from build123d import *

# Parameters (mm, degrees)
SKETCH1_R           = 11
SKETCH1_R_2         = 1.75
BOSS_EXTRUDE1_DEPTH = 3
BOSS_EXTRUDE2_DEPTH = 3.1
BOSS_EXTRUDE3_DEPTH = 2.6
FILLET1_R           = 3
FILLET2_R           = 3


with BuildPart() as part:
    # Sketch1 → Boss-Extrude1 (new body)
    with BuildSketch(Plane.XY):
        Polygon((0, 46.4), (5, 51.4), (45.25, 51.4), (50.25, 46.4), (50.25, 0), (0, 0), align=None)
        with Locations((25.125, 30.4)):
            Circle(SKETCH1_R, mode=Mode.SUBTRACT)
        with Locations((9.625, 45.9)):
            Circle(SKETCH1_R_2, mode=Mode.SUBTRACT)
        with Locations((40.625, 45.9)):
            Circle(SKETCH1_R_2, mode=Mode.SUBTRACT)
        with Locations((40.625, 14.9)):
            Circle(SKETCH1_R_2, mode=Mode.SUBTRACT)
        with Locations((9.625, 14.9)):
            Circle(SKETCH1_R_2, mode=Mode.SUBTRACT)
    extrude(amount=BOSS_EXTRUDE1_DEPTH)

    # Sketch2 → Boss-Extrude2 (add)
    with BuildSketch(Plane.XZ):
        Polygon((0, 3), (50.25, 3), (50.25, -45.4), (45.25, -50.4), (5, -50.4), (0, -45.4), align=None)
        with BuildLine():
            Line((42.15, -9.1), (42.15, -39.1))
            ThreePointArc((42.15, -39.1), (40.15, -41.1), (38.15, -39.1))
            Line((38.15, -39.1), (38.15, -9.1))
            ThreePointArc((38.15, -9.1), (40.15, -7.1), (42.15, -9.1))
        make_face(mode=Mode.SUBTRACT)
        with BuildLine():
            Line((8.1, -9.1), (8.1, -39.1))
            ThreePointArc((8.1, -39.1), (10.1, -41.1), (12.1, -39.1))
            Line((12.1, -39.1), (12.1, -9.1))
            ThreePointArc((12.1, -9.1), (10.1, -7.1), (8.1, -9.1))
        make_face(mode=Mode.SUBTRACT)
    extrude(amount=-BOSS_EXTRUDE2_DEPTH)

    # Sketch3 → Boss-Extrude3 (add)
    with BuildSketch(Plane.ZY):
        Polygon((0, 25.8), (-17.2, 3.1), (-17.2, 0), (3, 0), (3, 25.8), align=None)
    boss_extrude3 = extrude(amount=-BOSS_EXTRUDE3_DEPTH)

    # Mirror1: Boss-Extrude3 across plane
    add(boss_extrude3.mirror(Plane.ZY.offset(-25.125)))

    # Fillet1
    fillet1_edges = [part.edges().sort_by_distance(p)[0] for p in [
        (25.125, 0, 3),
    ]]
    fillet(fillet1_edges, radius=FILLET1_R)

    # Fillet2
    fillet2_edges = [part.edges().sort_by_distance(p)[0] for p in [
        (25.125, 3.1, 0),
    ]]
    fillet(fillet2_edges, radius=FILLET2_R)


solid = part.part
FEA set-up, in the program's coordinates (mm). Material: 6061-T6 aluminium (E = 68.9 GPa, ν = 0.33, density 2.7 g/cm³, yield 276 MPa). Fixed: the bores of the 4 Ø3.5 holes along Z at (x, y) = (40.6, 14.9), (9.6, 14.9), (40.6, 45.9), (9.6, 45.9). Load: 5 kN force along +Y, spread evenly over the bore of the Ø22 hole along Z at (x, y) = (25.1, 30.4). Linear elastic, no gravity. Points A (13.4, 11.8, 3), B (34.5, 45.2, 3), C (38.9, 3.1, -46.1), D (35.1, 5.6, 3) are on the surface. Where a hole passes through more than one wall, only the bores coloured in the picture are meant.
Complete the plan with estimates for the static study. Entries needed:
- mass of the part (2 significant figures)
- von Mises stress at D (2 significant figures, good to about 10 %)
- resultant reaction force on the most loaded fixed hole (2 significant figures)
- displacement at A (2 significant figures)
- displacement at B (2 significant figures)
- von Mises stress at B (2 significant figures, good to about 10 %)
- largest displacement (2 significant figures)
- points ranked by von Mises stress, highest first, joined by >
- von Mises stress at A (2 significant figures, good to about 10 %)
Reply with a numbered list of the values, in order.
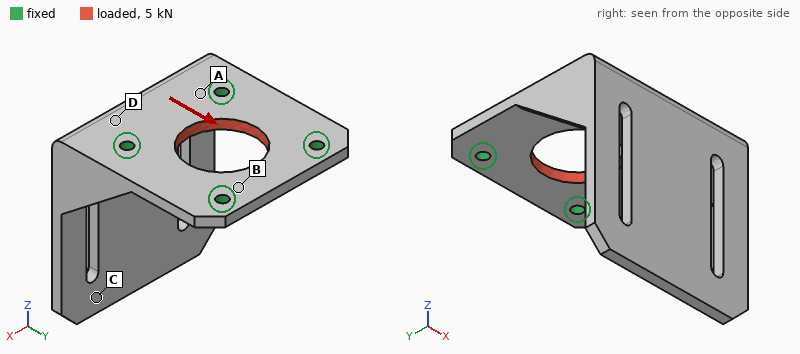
1. 39 g
2. 15 MPa
3. 1.3 kN
4. 2.6 µm
5. 6.8 µm
6. 34 MPa
7. 15 µm
8. B > A > D > C
9. 25 MPa
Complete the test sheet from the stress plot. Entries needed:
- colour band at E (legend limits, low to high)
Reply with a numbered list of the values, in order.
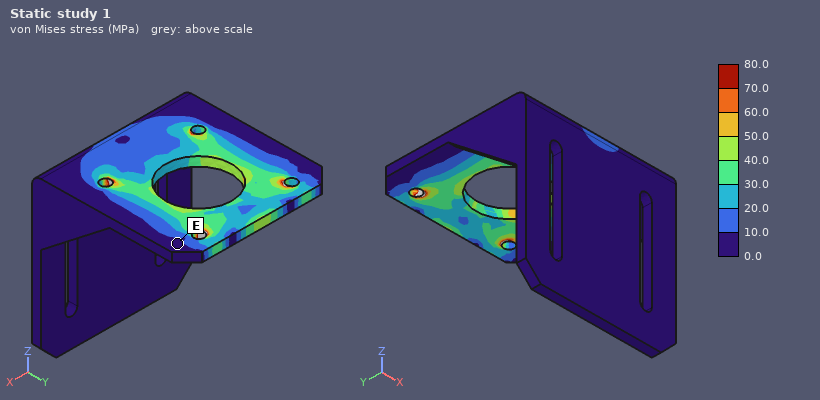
1. 0.0 to 10.0 MPa
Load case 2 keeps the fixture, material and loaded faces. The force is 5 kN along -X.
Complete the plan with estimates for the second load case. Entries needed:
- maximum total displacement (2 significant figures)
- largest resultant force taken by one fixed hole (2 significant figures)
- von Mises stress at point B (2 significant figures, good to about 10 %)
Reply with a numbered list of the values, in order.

1. 11 µm
2. 1.3 kN
3. 31 MPa
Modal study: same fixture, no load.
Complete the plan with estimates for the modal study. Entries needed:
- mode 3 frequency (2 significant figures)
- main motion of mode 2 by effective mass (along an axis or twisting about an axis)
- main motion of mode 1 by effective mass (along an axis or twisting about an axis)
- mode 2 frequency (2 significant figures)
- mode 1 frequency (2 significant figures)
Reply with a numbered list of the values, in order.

1. 3600 Hz
2. along X
3. along Y
4. 2200 Hz
5. 1100 Hz
